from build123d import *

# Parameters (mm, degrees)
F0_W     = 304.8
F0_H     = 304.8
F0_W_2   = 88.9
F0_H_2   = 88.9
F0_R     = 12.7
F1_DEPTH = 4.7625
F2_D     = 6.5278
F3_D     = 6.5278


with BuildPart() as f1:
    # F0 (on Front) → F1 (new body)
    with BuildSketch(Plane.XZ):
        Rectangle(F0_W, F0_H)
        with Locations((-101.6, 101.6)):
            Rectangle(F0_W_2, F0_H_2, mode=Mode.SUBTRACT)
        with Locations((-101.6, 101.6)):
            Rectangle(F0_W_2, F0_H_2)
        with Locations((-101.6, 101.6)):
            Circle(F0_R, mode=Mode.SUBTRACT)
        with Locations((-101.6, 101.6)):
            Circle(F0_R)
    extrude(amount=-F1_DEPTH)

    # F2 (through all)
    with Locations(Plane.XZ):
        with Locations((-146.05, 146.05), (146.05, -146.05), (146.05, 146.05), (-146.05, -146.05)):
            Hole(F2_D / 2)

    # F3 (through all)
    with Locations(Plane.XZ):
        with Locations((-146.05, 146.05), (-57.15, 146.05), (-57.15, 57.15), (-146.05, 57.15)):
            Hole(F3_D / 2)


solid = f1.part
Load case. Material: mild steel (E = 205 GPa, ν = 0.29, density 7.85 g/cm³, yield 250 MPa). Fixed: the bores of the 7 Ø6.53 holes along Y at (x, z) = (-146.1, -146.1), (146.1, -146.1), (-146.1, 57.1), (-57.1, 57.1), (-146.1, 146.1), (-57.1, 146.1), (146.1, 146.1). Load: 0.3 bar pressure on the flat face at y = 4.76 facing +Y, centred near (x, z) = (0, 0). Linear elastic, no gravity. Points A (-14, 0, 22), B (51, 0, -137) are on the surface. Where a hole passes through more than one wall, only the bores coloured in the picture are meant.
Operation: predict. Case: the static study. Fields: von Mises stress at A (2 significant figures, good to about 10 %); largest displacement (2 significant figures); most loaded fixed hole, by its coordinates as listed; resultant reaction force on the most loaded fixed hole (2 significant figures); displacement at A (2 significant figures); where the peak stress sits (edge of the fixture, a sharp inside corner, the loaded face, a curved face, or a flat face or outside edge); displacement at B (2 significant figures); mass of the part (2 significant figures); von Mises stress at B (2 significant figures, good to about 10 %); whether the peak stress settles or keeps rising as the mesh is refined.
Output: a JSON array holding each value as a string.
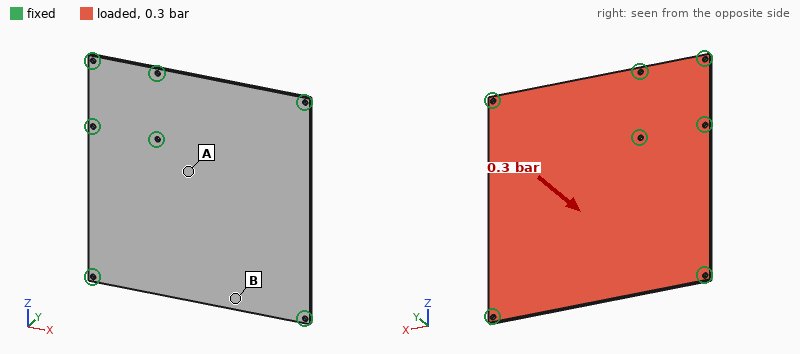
["14 MPa", "0.44 mm", "(-57.1, 57.1)", "1.2 kN", "0.19 mm", "edge of the fixture", "0.36 mm", "3.5 kg", "34 MPa", "keeps rising"]
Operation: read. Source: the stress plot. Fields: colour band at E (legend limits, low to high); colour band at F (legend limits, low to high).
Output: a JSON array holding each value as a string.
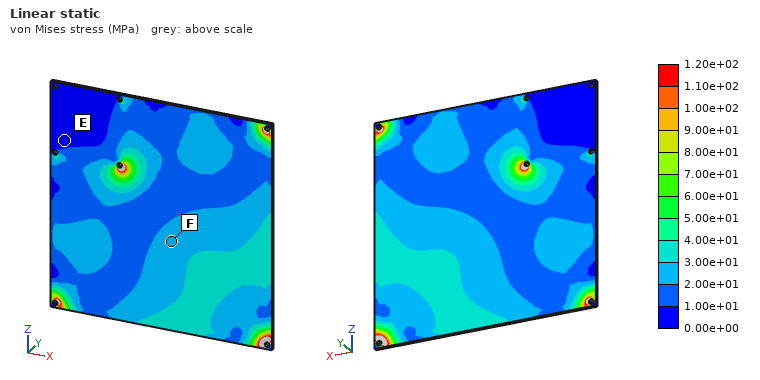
["0.00e+00 to 1.00e+01 MPa", "2.00e+01 to 3.00e+01 MPa"]
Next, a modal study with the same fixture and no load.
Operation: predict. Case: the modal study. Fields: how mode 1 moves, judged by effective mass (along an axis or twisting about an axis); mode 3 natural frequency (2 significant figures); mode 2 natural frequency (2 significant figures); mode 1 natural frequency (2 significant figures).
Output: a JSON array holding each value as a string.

["along Y", "560 Hz", "320 Hz", "240 Hz"]
